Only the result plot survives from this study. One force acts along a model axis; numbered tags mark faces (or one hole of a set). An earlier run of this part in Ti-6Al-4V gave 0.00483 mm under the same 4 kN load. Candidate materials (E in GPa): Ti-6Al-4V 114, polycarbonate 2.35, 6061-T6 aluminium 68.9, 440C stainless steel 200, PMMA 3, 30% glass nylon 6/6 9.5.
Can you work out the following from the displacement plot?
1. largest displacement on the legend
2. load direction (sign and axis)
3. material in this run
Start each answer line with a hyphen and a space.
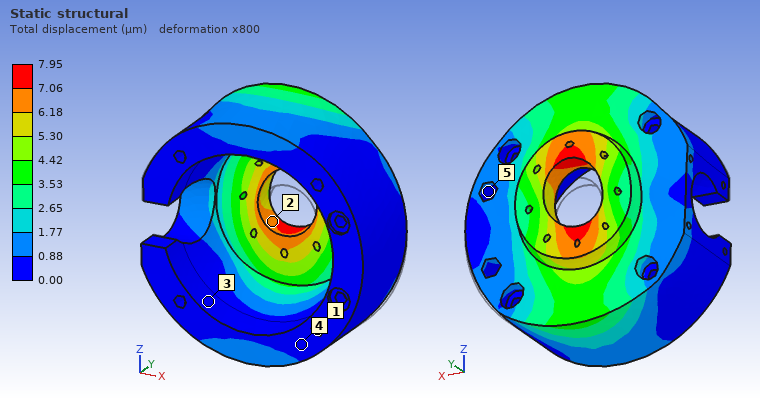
- 7.95 µm
- +Z
- 6061-T6 aluminium
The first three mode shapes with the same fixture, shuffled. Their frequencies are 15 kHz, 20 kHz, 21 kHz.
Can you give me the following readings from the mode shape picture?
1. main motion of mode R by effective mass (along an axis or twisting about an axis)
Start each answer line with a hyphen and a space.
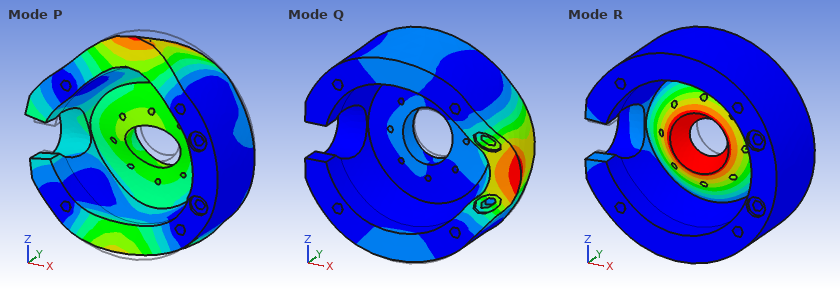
- along Y
